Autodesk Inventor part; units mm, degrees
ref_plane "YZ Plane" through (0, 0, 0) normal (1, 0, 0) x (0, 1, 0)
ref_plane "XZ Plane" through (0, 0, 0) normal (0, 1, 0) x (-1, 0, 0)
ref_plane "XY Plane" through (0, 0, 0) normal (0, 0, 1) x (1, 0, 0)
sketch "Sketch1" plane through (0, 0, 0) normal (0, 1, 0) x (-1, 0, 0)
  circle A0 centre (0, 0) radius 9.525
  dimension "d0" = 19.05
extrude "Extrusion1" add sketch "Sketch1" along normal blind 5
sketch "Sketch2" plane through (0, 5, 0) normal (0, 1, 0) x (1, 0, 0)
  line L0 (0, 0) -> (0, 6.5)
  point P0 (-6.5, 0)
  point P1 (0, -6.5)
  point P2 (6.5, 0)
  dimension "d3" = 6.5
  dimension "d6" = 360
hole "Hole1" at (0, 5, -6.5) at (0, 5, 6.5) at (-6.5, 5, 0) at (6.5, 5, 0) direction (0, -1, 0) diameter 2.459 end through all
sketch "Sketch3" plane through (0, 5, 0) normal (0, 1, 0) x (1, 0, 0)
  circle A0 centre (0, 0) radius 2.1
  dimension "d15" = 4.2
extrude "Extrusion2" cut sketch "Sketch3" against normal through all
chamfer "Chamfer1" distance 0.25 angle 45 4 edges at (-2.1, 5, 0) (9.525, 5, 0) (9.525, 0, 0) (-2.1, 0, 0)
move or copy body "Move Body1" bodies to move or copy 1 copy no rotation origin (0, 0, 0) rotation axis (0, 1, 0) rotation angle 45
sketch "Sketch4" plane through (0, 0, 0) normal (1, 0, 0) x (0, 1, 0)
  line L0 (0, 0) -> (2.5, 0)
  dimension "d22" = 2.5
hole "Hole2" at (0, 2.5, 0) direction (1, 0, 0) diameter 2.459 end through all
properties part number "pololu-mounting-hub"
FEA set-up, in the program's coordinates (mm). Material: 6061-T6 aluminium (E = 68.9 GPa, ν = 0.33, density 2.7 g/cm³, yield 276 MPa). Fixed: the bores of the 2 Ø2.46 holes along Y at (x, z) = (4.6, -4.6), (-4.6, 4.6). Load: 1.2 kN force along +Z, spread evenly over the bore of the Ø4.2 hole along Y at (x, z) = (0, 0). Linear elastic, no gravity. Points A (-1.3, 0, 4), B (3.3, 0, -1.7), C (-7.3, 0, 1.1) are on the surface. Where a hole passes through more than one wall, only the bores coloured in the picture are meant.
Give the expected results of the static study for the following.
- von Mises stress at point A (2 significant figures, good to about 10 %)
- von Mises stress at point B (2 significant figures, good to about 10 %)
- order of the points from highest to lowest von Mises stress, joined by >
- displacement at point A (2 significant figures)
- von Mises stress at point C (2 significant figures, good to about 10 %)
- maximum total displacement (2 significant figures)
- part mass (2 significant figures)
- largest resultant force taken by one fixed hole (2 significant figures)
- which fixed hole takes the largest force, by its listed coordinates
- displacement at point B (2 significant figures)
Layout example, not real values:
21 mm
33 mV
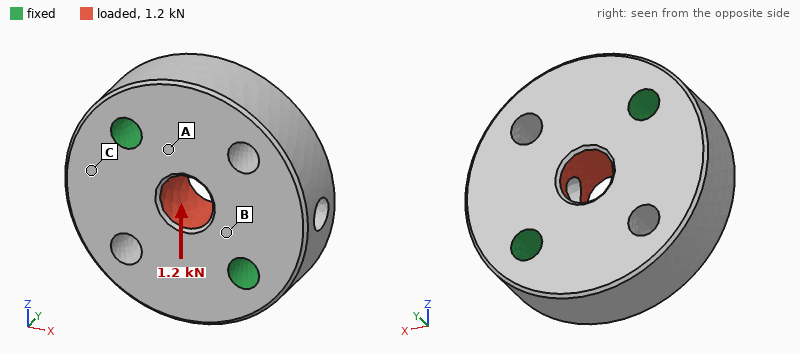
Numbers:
15 MPa
24 MPa
B > A > C
1.4 µm
5.7 MPa
2.4 µm
3.3 g
660 N
(-4.6, 4.6)
0.96 µm
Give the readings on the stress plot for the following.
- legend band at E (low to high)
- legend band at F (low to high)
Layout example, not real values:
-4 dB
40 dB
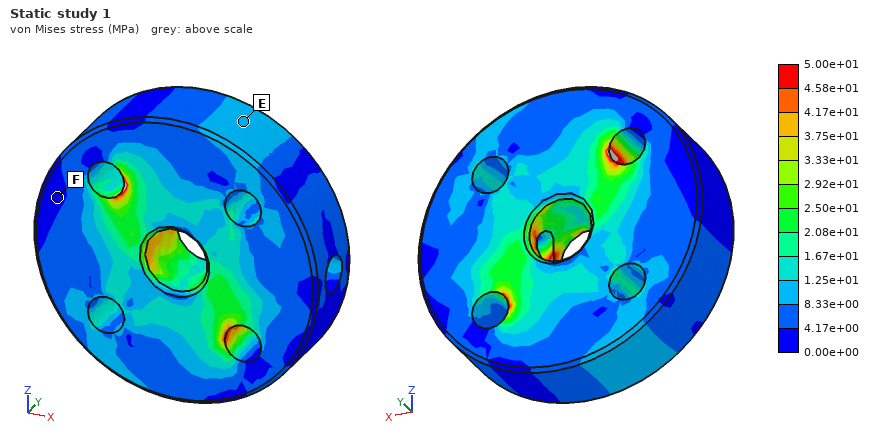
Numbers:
8.33e+00 to 1.25e+01 MPa
0.00e+00 to 4.17e+00 MPa
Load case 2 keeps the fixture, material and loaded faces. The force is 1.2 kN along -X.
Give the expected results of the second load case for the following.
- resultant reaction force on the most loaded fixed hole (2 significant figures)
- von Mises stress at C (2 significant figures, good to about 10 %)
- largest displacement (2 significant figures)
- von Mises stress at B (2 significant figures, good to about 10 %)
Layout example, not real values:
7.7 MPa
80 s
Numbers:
610 N
8.5 MPa
2.4 µm
15 MPa
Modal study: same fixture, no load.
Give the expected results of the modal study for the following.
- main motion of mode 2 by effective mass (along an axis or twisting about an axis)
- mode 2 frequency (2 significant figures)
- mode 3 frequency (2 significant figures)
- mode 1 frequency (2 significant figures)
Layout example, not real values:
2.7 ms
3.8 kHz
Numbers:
along Y
45 kHz
78 kHz
39 kHz
